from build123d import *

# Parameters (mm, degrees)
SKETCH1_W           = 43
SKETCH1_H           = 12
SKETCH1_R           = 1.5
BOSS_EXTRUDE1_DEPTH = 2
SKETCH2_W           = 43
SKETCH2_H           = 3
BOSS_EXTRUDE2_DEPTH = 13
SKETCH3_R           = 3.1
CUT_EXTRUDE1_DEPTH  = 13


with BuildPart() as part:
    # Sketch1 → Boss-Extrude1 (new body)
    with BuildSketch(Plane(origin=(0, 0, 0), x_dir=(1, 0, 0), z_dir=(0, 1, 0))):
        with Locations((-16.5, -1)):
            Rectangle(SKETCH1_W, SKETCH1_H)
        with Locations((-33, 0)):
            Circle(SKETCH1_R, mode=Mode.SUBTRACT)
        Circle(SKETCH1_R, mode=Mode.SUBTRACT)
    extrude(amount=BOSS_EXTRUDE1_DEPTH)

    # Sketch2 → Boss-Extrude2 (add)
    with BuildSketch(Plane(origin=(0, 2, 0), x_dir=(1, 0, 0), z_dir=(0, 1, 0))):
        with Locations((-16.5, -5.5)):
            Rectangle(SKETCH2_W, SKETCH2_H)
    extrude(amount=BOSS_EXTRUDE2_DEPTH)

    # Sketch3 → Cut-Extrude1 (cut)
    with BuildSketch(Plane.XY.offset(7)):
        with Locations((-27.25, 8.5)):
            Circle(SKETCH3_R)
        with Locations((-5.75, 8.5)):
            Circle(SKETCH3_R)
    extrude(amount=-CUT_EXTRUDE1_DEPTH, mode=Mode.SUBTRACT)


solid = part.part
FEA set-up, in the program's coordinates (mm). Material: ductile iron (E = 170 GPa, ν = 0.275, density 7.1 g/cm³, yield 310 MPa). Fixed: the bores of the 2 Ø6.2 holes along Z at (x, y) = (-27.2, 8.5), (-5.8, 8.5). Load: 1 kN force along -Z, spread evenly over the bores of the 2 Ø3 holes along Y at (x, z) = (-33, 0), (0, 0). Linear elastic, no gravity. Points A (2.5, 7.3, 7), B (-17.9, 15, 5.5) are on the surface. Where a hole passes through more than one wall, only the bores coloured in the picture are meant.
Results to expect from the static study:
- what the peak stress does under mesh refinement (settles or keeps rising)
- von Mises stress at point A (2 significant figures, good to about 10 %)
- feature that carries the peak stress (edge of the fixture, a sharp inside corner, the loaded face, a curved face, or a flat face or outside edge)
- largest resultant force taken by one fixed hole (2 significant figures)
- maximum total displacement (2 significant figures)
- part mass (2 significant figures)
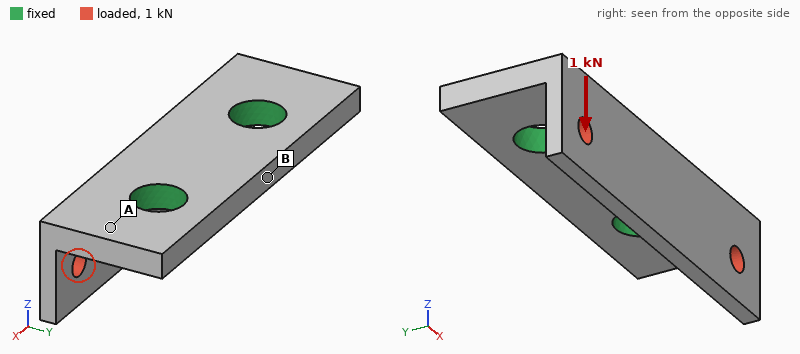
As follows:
keeps rising
34 MPa
edge of the fixture
520 N
19 µm
18 g
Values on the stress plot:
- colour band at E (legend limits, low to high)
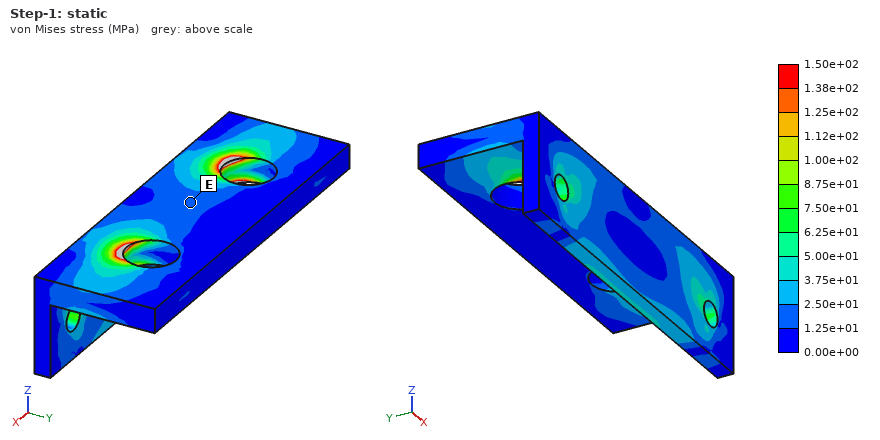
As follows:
1.25e+01 to 2.50e+01 MPa
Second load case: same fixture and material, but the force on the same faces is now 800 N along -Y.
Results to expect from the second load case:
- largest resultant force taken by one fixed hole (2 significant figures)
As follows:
400 N
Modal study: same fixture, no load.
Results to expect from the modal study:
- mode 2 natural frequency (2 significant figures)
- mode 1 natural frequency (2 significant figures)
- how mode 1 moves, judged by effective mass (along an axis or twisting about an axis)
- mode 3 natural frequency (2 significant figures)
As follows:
13 kHz
12 kHz
along Y
20 kHz
